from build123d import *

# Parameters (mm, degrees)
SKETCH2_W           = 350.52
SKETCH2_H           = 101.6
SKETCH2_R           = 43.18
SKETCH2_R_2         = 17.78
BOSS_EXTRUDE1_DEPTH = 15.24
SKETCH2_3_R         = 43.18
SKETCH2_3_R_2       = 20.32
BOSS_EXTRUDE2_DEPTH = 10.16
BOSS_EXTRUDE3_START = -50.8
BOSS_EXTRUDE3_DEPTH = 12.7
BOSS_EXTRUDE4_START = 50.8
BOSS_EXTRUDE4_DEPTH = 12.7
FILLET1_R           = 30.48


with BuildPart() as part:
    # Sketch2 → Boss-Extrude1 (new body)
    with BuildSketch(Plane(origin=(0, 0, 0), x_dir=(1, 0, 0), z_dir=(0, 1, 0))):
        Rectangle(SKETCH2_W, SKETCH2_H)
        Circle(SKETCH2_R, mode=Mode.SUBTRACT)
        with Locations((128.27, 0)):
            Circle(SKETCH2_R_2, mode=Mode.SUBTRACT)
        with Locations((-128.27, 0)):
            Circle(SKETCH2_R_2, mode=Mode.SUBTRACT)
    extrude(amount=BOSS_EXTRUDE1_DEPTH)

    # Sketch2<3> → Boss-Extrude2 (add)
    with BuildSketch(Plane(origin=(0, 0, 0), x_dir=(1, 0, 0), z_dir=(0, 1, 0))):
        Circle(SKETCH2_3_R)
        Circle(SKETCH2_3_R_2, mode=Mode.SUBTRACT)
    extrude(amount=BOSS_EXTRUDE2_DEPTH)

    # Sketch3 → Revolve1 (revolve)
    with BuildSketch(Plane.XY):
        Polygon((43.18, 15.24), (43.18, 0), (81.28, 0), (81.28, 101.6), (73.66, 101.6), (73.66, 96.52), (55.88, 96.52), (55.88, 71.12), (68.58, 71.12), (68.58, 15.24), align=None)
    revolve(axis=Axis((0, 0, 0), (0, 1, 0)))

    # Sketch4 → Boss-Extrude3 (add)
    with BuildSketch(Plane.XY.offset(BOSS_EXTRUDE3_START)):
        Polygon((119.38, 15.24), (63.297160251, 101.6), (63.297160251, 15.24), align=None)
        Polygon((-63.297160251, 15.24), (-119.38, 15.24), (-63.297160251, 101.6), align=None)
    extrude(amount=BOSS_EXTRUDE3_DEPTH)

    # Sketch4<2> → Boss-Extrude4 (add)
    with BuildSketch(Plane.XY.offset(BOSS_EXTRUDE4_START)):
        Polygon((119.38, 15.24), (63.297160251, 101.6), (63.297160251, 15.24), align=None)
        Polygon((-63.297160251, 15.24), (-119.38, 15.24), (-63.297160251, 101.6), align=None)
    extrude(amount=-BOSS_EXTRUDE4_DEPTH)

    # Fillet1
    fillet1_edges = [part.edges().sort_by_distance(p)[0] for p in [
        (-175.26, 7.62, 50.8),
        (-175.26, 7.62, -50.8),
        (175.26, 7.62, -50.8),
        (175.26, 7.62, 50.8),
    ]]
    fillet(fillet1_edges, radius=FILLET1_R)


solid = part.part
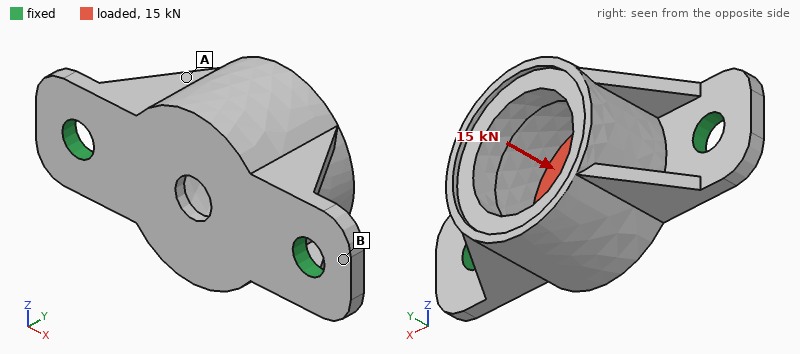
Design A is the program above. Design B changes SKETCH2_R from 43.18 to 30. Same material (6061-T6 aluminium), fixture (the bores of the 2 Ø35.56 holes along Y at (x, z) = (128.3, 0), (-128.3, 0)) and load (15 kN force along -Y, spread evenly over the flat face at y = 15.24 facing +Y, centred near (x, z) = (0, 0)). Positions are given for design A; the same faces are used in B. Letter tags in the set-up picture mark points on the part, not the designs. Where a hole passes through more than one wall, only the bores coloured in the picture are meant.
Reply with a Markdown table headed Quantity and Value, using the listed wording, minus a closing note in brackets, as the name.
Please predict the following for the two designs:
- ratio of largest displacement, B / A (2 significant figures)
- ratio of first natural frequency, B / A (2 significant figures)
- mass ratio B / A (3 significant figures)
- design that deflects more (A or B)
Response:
| Quantity | Value |
|---|---|
| ratio of largest displacement, B / A | 1.1 |
| ratio of first natural frequency, B / A | 1.00 |
| mass ratio B / A | 1.01 |
| design that deflects more | B |
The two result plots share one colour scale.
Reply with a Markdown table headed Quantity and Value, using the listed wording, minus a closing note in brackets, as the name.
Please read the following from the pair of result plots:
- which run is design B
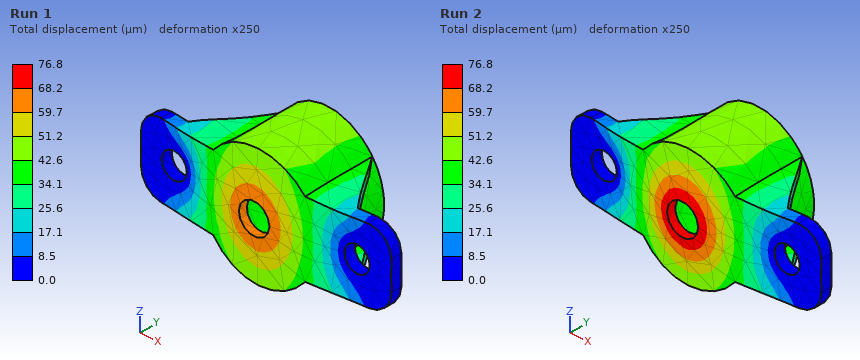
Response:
| Quantity | Value |
|---|---|
| which run is design B | Run 2 |
